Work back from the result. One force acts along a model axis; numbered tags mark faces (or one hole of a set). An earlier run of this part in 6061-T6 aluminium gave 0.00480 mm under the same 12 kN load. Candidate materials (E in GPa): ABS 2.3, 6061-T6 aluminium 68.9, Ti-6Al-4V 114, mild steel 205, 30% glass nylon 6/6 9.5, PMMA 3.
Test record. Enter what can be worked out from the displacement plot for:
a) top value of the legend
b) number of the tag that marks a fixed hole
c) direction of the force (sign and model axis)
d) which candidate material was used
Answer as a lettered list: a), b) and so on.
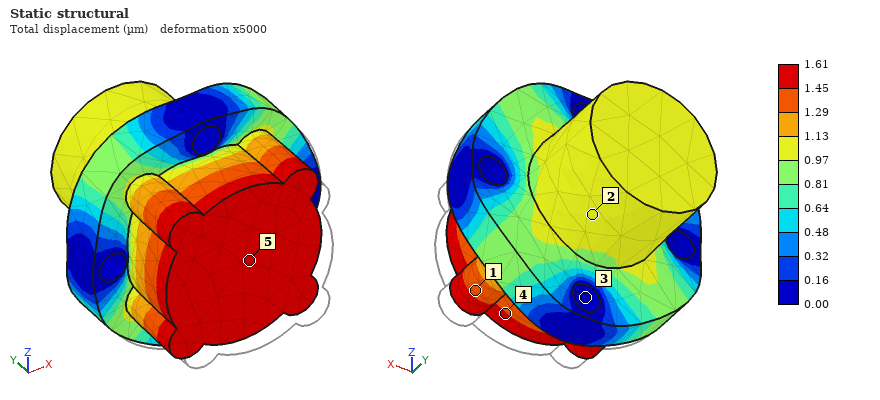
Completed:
a) 1.61 µm
b) 3
c) +Y
d) mild steel
